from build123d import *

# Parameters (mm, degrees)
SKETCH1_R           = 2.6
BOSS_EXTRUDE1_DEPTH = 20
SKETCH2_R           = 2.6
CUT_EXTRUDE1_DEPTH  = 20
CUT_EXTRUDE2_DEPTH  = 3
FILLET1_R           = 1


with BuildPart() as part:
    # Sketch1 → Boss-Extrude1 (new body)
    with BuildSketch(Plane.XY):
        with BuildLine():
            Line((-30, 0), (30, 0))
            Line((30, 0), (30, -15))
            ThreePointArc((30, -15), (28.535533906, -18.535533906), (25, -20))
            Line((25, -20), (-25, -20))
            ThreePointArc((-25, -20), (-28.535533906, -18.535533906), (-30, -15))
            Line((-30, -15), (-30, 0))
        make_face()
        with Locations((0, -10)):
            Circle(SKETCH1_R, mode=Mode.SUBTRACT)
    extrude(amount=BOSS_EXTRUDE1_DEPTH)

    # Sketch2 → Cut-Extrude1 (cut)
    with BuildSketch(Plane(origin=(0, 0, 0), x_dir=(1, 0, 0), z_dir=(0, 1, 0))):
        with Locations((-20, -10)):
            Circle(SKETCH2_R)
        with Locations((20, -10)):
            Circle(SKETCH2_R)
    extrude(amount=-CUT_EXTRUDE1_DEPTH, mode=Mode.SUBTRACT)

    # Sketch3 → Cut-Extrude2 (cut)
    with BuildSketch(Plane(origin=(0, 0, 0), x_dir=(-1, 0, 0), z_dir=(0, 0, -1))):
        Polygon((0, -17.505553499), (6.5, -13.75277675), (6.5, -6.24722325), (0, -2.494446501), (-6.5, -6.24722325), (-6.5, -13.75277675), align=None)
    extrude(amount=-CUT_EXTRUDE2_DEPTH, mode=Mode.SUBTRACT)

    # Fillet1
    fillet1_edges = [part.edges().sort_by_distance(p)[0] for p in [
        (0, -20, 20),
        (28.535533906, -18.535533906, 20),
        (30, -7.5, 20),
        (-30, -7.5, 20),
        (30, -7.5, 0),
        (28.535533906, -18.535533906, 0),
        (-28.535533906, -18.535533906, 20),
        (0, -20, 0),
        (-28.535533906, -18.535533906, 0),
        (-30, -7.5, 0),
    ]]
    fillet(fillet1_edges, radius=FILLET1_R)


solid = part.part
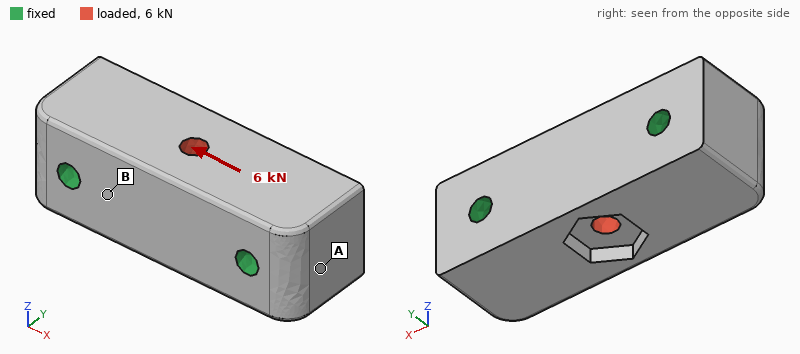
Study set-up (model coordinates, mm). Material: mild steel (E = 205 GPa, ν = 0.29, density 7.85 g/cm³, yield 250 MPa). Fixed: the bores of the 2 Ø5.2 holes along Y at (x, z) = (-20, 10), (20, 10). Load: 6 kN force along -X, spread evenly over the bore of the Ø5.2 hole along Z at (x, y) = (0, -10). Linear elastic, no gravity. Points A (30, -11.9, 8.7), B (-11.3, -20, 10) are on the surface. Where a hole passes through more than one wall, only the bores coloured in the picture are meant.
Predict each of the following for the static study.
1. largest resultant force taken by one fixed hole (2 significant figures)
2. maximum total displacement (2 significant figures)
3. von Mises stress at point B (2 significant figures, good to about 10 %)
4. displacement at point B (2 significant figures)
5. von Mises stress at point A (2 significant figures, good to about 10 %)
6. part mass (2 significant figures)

3.0 kN
1.2 µm
9.0 MPa
0.39 µm
3.6 MPa
170 g
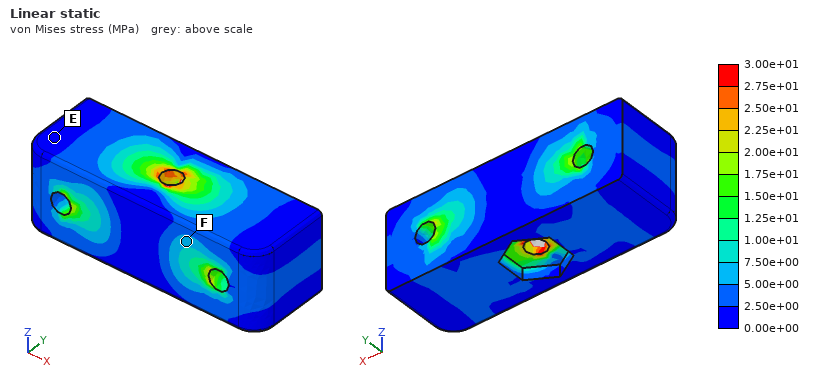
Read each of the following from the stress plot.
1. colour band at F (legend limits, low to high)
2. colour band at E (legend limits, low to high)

5.00e+00 to 7.50e+00 MPa
0.00e+00 to 2.50e+00 MPa
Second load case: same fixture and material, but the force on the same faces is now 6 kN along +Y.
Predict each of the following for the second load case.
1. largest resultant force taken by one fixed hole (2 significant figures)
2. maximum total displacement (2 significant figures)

3.0 kN
3.5 µm
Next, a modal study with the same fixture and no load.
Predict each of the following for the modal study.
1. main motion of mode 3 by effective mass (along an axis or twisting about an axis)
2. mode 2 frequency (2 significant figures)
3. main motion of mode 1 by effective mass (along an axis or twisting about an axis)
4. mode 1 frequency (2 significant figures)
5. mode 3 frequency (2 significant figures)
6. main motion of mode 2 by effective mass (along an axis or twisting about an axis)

twisting about X
33 kHz
along Z
26 kHz
37 kHz
along Y
